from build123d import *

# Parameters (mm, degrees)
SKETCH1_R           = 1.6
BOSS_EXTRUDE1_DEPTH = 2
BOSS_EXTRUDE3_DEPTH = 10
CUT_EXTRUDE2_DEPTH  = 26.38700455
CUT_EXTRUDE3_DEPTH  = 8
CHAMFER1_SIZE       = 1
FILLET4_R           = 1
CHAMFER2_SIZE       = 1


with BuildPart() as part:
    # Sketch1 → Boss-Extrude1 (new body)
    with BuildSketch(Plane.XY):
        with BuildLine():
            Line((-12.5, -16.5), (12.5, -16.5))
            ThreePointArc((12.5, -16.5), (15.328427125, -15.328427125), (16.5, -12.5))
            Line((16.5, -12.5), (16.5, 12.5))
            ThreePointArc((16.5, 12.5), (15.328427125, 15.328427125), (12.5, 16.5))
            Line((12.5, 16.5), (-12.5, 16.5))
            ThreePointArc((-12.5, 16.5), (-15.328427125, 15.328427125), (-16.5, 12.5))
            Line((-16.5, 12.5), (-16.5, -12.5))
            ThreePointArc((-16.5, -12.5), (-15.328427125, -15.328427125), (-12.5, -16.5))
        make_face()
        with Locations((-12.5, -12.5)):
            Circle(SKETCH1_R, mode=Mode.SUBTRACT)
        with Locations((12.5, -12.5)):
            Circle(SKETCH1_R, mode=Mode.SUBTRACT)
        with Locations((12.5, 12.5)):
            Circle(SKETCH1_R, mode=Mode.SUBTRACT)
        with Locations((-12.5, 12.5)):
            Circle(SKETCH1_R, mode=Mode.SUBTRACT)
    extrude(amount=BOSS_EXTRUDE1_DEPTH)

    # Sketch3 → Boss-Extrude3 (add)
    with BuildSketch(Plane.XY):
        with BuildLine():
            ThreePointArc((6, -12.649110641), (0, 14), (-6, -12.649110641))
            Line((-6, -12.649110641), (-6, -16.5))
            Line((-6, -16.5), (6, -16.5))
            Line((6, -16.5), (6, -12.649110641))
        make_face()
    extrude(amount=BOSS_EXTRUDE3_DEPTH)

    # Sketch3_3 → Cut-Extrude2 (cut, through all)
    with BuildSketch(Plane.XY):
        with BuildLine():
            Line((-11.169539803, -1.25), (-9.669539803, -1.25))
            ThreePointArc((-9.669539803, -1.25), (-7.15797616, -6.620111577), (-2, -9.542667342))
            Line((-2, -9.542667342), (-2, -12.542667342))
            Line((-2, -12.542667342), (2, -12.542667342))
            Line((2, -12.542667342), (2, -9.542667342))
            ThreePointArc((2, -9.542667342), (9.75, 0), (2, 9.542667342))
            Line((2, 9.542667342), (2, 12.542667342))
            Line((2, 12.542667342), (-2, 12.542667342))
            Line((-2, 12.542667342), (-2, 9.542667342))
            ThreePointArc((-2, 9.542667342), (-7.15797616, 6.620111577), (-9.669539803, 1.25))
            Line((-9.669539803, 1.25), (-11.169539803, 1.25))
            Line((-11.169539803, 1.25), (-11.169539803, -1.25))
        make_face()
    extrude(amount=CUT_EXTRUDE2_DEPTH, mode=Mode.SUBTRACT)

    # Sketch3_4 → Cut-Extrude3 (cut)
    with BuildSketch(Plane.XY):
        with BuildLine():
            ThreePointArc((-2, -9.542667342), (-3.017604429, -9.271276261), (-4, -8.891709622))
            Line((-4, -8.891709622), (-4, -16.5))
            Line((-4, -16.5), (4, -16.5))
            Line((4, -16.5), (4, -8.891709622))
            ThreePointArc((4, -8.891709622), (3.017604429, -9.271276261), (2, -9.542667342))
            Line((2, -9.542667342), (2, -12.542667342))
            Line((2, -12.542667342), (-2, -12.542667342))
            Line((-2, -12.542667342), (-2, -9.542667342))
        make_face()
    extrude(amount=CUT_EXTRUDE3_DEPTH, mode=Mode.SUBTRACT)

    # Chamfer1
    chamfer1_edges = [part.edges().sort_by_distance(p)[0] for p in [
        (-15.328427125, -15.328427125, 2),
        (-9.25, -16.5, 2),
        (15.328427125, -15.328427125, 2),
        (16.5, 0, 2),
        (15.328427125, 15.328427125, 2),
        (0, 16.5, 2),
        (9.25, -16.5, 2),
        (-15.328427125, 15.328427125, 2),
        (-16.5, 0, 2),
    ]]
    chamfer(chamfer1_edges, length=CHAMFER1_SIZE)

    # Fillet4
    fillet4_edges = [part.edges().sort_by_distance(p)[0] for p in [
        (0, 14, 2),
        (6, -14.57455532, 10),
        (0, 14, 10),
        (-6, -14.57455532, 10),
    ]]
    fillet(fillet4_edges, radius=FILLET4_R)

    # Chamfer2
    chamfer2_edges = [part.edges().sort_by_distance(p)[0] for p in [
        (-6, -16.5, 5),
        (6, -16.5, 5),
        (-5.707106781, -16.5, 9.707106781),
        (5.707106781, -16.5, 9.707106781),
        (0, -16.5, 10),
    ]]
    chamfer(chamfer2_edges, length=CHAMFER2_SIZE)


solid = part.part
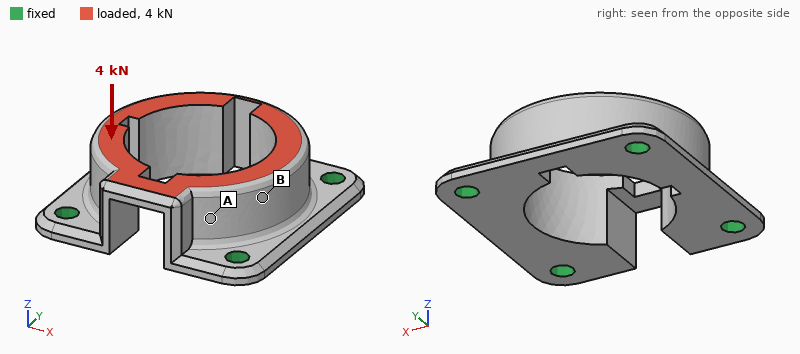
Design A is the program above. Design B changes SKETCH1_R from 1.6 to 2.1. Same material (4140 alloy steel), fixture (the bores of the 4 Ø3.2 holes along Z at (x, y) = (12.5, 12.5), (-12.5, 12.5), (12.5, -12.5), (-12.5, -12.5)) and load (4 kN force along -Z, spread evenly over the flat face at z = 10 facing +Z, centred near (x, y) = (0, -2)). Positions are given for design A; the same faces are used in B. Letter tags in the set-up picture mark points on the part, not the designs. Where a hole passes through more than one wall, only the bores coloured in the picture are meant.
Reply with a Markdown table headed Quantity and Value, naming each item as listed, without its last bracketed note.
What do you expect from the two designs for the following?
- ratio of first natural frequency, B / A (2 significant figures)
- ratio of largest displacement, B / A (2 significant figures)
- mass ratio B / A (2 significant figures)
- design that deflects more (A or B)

| Quantity | Value |
|---|---|
| ratio of first natural frequency, B / A | 1.1 |
| ratio of largest displacement, B / A | 0.83 |
| mass ratio B / A | 0.99 |
| design that deflects more | A |
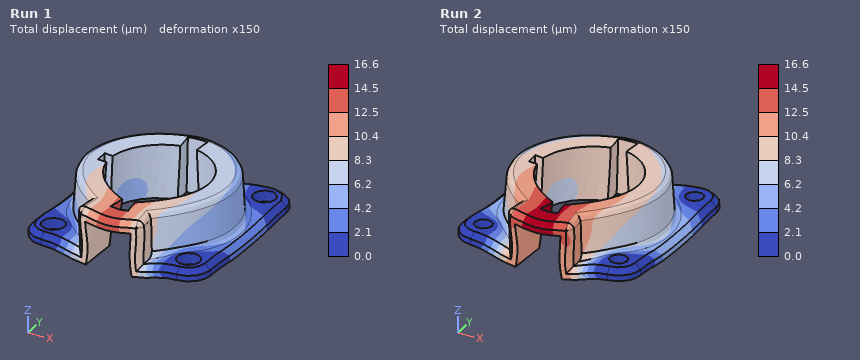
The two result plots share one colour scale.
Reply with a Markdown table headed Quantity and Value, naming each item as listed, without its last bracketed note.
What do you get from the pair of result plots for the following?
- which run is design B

| Quantity | Value |
|---|---|
| which run is design B | Run 1 |
